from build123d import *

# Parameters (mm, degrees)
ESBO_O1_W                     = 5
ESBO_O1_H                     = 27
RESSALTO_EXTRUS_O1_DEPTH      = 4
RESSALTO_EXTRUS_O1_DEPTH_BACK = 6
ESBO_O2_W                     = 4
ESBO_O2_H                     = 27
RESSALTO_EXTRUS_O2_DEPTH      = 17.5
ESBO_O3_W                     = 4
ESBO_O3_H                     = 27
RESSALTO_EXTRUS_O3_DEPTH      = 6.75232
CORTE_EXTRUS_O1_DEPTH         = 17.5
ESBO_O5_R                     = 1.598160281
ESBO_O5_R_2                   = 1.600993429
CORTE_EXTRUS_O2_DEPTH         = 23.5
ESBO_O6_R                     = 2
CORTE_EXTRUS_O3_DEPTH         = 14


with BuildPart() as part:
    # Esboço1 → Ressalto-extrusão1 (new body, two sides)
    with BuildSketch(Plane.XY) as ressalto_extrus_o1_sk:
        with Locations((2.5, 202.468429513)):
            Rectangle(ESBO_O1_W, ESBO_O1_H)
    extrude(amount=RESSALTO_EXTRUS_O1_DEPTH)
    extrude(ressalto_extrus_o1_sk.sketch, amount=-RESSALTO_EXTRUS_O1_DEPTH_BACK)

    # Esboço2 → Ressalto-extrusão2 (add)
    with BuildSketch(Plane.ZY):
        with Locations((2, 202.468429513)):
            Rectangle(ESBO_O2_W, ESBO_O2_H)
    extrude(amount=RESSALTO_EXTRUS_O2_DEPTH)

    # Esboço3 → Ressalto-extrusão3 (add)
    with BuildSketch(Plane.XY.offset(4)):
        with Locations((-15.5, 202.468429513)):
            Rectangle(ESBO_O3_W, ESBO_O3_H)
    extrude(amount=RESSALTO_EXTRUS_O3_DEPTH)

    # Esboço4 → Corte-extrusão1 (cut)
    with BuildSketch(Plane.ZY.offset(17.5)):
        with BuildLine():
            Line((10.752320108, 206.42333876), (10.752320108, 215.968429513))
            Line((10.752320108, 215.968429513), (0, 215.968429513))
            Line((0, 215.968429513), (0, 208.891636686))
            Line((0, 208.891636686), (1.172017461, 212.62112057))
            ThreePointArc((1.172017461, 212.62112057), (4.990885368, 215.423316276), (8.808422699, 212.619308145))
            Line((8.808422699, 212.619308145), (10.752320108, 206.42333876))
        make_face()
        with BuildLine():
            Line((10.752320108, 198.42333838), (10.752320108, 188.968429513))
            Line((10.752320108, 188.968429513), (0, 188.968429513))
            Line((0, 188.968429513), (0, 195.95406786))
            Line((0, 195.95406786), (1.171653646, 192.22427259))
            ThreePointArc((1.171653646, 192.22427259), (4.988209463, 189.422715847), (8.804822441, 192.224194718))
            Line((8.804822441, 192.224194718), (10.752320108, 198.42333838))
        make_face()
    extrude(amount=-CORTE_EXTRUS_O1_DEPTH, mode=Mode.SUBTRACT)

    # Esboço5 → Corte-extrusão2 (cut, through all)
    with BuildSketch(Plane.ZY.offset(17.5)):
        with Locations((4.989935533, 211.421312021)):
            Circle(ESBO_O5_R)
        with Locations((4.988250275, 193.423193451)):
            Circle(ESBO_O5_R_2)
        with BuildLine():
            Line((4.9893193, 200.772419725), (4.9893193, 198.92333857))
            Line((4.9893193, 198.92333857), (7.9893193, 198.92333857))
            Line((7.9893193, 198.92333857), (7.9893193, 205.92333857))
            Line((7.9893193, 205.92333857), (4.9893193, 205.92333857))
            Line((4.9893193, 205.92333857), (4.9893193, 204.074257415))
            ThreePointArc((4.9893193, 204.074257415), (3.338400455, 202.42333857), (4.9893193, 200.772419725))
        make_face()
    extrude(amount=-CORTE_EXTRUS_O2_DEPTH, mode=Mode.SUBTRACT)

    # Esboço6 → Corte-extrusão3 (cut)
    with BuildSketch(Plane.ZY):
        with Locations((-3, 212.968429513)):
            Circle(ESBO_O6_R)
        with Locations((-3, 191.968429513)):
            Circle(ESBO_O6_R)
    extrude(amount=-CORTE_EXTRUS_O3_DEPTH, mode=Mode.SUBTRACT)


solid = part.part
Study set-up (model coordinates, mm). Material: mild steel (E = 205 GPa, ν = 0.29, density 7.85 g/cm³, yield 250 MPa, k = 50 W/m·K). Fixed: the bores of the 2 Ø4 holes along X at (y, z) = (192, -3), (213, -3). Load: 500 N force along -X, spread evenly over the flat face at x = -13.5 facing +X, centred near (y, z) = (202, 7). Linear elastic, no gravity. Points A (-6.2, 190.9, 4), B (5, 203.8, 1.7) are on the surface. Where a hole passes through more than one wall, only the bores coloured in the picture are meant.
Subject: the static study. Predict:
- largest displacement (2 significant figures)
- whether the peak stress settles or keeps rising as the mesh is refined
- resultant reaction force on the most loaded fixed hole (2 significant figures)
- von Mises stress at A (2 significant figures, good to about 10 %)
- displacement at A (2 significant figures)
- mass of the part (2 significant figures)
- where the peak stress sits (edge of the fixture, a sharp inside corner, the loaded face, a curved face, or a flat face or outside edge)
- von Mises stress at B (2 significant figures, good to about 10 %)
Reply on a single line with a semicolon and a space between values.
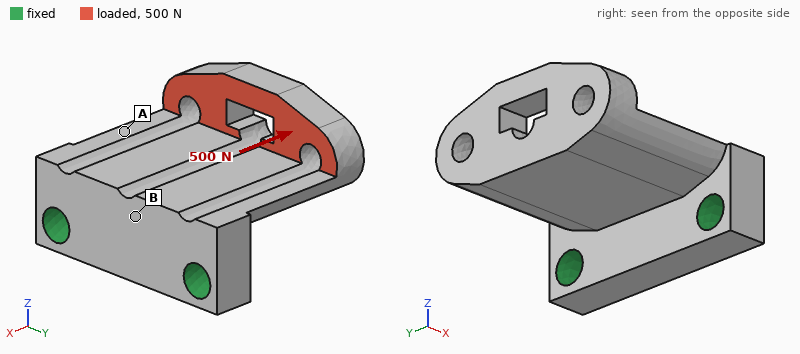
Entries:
41 µm; keeps rising; 250 N; 57 MPa; 7.3 µm; 24 g; edge of the fixture; 9.0 MPa
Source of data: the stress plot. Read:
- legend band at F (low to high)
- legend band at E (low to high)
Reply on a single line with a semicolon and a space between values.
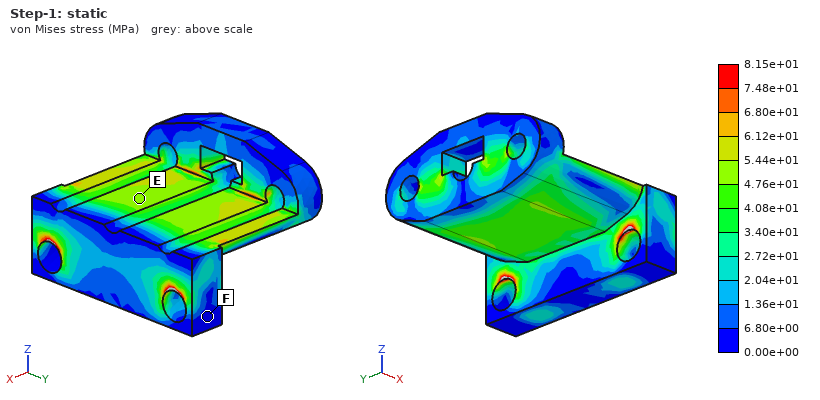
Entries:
0.00e+00 to 6.80e+00 MPa; 4.76e+01 to 5.44e+01 MPa
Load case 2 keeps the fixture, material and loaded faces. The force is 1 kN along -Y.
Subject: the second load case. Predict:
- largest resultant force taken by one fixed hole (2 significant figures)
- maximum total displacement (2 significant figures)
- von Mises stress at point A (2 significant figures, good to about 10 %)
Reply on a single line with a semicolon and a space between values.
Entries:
1.0 kN; 36 µm; 50 MPa
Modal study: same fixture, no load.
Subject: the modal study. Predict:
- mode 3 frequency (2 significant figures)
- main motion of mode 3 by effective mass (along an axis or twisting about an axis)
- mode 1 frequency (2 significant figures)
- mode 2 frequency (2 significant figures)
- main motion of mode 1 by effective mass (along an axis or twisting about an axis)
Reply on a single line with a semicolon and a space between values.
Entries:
17 kHz; along Y; 5100 Hz; 11 kHz; along Z
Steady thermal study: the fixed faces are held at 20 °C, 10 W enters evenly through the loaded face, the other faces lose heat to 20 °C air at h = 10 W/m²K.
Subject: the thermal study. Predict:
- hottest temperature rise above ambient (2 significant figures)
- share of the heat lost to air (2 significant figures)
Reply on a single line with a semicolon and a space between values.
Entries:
68 K; 5.6 %
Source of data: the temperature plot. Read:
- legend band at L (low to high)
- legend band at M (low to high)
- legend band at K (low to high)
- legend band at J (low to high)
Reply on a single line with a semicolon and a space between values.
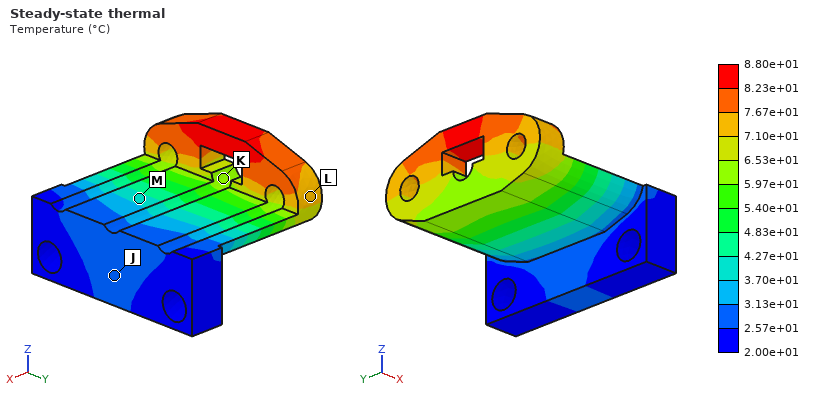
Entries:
7.10e+01 to 7.67e+01 °C; 3.70e+01 to 4.27e+01 °C; 5.97e+01 to 6.53e+01 °C; 2.57e+01 to 3.13e+01 °C
